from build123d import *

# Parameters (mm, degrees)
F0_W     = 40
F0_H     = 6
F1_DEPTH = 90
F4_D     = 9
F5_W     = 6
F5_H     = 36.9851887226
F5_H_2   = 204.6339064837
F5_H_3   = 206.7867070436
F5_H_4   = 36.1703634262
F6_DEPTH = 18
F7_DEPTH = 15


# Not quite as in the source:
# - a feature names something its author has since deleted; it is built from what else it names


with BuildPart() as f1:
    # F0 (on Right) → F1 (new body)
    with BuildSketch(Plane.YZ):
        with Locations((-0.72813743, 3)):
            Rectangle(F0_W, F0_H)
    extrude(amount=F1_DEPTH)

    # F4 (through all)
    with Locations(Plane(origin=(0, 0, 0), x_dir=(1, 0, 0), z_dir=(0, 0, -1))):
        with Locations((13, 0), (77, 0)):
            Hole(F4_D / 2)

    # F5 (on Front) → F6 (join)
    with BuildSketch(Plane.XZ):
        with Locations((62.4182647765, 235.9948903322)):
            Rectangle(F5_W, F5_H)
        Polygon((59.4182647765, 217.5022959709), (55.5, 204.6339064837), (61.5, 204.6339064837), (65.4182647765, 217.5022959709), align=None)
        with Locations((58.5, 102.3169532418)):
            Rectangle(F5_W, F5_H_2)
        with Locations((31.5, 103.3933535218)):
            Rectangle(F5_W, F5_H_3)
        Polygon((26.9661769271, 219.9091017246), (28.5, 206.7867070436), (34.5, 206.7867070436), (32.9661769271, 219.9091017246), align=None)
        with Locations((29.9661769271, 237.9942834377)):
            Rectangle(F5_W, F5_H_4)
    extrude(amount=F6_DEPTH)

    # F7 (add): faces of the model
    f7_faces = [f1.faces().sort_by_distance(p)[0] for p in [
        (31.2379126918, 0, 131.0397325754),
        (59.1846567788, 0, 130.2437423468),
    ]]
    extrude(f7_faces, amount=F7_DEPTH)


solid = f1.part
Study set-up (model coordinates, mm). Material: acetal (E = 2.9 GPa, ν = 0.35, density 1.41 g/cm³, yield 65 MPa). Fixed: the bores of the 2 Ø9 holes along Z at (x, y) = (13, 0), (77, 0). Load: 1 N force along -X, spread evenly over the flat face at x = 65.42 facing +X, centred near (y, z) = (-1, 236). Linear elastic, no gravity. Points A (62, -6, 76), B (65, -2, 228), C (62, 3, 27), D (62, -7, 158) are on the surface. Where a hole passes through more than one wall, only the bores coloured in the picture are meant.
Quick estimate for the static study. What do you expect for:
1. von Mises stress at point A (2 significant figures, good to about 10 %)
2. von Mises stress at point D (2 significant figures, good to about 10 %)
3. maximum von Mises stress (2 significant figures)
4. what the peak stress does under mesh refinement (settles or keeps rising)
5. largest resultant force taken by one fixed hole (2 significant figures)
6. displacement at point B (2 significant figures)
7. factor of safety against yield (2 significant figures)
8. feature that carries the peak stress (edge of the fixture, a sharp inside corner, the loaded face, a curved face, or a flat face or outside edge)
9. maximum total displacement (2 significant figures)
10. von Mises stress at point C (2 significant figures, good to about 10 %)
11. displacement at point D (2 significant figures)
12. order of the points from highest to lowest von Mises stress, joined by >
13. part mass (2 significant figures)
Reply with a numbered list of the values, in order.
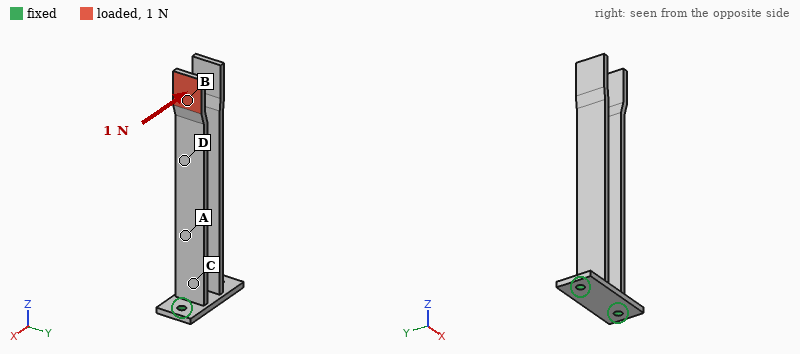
1. 0.81 MPa
2. 0.40 MPa
3. 1.1 MPa
4. settles
5. 4.6 N
6. 2.3 mm
7. 58
8. a flat face or outside edge
9. 2.8 mm
10. 1.0 MPa
11. 1.3 mm
12. C > A > D > B
13. 170 g
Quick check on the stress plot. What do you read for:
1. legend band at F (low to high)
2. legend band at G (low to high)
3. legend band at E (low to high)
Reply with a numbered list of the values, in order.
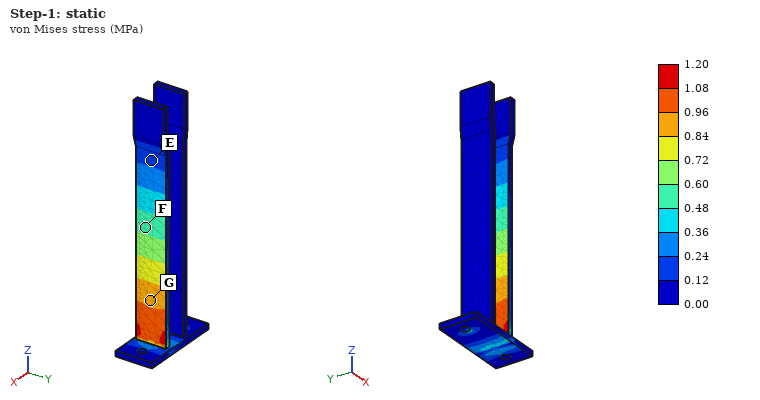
1. 0.48 to 0.60 MPa
2. 0.84 to 0.96 MPa
3. 0.12 to 0.24 MPa
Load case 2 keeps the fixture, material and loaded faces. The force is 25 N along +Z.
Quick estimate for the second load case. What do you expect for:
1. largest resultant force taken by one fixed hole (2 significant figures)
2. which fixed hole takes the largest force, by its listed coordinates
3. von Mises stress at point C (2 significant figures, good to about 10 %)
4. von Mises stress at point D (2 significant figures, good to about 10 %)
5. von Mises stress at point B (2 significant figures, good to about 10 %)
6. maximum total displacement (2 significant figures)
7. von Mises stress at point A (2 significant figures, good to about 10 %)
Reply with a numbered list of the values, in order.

1. 23 N
2. (77, 0)
3. 0.97 MPa
4. 1.00 MPa
5. 0.37 MPa
6. 3.0 mm
7. 1.00 MPa
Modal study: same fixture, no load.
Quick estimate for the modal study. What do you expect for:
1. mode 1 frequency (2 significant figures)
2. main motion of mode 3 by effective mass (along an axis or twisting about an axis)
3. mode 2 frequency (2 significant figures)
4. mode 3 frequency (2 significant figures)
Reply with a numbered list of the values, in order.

1. 21 Hz
2. along Y
3. 22 Hz
4. 58 Hz
